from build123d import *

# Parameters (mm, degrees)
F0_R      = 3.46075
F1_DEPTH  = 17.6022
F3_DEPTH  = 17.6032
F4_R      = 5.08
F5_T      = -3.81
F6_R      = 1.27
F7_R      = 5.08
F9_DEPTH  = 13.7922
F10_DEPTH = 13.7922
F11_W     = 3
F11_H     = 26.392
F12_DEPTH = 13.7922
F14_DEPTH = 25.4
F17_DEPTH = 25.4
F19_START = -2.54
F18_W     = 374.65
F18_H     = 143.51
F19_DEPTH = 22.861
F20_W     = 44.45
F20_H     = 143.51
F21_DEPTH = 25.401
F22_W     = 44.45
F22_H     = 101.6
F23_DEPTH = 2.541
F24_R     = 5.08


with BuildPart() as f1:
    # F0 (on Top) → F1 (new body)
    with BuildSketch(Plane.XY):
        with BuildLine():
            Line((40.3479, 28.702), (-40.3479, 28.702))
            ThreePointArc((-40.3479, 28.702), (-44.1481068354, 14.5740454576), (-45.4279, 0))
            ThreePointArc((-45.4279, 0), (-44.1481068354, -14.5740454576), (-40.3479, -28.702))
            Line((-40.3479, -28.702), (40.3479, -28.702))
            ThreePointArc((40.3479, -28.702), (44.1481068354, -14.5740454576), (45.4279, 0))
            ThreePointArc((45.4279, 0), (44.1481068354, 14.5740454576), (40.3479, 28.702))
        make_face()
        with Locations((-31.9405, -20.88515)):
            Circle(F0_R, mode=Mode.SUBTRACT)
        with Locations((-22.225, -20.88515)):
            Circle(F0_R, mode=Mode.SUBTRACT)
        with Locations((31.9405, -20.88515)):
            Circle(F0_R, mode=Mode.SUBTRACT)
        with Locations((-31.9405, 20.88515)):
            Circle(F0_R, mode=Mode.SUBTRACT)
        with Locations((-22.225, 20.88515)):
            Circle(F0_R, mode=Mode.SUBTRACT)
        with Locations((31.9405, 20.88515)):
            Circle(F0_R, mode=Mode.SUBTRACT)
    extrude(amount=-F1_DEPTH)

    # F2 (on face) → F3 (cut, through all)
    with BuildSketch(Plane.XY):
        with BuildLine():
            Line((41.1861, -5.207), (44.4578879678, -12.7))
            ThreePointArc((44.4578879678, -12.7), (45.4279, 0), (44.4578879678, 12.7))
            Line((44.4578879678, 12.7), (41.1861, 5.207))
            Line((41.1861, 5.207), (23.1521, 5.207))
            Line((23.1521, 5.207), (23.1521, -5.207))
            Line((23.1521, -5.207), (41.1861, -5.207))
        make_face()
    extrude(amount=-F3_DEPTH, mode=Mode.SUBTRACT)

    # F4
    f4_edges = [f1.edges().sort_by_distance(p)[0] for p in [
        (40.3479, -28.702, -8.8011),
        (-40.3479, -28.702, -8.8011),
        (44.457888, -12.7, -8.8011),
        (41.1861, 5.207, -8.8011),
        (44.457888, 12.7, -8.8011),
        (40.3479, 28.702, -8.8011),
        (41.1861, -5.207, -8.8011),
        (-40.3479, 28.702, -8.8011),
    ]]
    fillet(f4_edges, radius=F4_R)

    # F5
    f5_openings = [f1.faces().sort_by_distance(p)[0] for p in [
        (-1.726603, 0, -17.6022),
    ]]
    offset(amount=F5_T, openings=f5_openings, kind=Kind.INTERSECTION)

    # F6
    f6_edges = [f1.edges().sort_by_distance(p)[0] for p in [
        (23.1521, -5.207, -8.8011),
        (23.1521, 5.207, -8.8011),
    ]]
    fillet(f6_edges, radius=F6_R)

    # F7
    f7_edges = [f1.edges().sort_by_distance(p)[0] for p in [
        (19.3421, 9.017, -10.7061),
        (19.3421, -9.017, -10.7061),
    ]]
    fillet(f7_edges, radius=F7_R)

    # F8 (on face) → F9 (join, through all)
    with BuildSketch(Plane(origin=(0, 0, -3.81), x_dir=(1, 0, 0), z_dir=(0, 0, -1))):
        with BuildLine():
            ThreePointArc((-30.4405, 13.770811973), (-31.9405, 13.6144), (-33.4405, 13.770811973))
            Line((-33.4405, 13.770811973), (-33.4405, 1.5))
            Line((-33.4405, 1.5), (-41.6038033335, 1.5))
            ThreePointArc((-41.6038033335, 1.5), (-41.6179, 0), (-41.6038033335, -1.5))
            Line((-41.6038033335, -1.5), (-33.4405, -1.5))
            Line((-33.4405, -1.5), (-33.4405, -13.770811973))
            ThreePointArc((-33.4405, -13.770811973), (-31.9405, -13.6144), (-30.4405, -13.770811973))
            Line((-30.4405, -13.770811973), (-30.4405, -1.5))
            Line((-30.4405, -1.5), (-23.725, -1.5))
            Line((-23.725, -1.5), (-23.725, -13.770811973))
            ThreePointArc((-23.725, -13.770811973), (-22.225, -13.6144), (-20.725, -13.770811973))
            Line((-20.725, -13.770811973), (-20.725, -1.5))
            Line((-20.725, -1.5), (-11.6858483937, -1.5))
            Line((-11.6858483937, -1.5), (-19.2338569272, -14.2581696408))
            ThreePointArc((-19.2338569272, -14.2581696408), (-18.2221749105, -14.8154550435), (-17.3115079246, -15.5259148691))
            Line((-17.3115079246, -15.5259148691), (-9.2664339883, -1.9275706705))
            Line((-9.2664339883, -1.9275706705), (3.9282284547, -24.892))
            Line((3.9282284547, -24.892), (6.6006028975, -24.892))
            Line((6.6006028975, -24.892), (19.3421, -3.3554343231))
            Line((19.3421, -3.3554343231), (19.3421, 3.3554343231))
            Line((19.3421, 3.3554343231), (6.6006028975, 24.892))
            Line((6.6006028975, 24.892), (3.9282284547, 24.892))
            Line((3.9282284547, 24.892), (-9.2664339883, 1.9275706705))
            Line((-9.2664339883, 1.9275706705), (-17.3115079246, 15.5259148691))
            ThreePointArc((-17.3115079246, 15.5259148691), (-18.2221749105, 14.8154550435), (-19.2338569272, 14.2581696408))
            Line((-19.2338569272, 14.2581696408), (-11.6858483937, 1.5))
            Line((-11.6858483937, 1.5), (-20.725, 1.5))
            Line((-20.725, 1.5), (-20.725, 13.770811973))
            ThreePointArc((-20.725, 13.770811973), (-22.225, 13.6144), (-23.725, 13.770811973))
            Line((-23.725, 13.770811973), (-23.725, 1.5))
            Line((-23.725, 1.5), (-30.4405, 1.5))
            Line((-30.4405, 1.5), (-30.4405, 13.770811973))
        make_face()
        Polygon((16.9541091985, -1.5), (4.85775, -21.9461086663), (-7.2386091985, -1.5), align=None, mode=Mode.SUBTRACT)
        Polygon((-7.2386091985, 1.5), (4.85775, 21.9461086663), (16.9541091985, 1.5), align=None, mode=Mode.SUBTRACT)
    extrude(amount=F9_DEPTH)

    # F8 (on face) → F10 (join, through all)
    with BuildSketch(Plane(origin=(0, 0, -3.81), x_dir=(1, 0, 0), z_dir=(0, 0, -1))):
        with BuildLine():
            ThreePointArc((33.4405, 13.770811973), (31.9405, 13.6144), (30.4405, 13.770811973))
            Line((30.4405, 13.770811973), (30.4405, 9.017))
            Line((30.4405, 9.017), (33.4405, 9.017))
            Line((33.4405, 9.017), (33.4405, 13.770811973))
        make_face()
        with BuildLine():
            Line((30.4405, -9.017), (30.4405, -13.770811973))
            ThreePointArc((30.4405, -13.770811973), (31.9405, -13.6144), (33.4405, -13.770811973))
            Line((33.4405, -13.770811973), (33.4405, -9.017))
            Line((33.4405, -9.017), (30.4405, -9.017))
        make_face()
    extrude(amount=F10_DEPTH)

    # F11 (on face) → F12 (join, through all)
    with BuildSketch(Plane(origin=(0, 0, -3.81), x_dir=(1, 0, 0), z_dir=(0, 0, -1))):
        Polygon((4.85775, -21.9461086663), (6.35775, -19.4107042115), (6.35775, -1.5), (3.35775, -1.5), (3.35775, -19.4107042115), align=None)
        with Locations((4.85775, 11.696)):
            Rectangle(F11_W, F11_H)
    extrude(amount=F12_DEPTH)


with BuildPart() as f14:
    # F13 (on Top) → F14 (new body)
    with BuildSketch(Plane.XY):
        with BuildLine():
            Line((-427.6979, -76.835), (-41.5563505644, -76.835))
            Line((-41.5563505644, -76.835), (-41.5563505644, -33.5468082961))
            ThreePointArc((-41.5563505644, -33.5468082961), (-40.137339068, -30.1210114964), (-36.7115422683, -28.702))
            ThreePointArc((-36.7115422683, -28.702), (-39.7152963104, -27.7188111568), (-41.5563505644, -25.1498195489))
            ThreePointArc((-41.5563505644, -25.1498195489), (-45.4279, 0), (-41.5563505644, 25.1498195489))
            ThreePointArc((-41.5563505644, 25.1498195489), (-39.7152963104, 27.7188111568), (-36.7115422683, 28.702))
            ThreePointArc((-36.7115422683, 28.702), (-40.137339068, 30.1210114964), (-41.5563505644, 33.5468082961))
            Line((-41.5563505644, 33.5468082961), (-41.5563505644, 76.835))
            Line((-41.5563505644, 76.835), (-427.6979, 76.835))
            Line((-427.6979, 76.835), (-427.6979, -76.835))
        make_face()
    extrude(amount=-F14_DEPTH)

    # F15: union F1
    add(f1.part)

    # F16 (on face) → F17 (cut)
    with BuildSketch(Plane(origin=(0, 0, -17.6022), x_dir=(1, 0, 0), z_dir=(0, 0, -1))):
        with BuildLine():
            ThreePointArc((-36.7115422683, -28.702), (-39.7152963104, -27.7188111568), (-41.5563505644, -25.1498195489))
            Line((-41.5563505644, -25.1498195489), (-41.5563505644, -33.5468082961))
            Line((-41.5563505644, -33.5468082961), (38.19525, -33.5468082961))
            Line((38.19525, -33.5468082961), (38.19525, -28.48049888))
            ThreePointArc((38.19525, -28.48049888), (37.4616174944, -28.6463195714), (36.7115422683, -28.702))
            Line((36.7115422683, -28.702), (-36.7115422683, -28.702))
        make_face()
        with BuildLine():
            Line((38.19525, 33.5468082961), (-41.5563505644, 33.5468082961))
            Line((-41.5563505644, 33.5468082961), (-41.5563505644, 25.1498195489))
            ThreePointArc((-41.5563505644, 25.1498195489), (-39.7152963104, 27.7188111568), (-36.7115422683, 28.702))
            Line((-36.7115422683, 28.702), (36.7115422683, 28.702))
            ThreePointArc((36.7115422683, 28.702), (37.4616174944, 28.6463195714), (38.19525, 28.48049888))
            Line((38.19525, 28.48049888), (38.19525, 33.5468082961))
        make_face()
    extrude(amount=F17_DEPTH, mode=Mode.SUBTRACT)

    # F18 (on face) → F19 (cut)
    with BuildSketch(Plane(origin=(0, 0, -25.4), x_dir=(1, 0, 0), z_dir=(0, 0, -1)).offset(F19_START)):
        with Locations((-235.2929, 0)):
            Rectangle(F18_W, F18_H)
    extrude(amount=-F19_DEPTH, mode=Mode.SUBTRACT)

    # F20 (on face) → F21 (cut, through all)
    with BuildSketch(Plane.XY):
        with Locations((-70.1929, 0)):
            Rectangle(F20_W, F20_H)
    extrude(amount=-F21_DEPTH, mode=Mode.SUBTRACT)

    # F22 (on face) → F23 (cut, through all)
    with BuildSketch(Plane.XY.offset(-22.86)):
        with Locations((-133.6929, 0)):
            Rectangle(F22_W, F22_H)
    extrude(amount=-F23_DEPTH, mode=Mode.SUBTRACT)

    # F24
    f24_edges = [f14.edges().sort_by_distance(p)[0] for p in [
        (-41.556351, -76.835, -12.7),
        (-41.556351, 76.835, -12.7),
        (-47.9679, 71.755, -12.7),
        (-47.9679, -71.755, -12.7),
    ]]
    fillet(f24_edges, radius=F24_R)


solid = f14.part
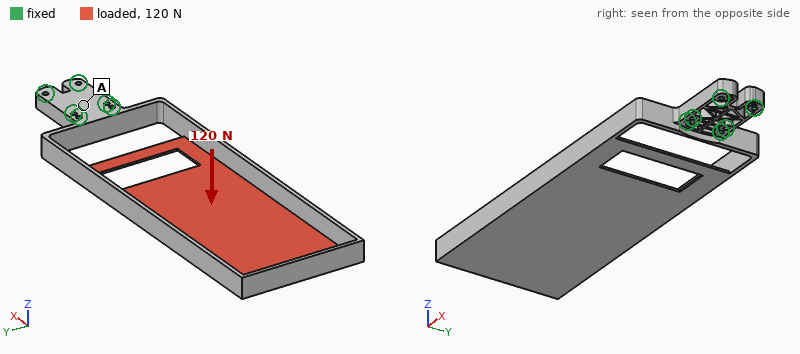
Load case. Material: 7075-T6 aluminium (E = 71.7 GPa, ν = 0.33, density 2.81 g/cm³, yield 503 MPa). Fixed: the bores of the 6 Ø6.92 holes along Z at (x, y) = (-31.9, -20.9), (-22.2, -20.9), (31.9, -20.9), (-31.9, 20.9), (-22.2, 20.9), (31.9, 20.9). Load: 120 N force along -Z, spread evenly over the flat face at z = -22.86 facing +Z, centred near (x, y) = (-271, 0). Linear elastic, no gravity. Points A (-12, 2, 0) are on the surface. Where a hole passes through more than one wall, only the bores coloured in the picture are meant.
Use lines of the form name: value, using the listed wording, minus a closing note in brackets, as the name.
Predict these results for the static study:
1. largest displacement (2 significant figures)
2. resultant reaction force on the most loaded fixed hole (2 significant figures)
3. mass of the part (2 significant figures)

largest displacement: 4.9 mm
resultant reaction force on the most loaded fixed hole: 140 N
mass of the part: 840 g
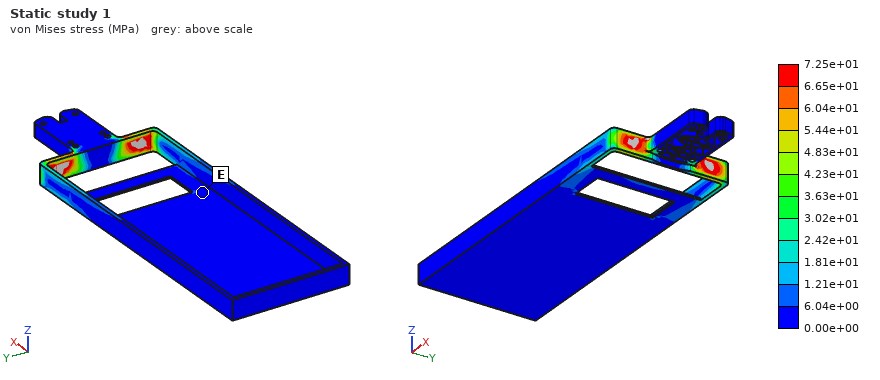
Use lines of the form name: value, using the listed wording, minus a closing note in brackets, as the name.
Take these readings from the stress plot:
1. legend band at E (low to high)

legend band at E: 0.00e+00 to 6.04e+00 MPa
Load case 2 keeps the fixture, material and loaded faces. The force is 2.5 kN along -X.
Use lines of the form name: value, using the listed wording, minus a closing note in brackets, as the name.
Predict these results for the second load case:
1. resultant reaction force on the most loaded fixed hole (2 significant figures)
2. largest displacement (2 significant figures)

resultant reaction force on the most loaded fixed hole: 2.7 kN
largest displacement: 5.0 mm
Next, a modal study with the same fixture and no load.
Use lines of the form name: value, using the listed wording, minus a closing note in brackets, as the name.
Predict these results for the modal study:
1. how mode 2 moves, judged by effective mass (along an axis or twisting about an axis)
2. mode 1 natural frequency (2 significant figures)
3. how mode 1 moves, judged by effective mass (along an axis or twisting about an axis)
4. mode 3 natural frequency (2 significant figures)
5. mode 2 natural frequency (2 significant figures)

how mode 2 moves, judged by effective mass: along Y
mode 1 natural frequency: 37 Hz
how mode 1 moves, judged by effective mass: along Z
mode 3 natural frequency: 100 Hz
mode 2 natural frequency: 71 Hz
